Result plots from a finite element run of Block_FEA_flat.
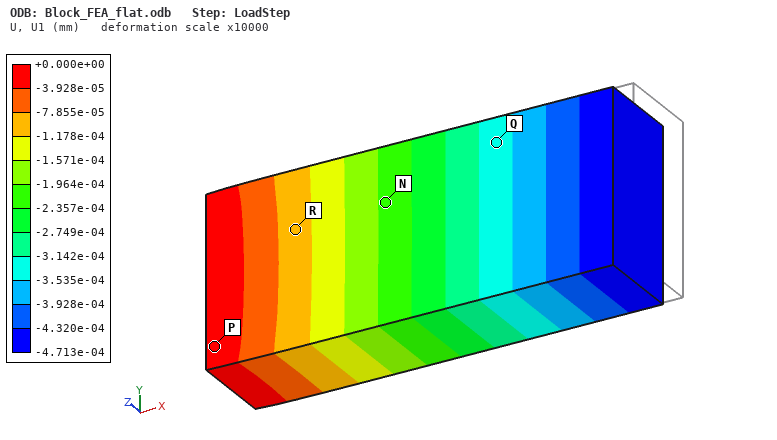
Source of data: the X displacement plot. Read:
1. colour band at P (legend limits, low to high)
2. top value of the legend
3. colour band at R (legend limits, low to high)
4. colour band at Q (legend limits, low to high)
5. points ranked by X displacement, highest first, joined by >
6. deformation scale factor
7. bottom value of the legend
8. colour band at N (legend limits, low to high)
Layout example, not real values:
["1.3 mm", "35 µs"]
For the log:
["-3.928e-05 to +0.000e+00 mm", "+0.000e+00 mm", "-1.178e-04 to -7.855e-05 mm", "-3.535e-04 to -3.142e-04 mm", "P > R > N > Q", "10000", "-4.713e-04 mm", "-2.357e-04 to -1.964e-04 mm"]
